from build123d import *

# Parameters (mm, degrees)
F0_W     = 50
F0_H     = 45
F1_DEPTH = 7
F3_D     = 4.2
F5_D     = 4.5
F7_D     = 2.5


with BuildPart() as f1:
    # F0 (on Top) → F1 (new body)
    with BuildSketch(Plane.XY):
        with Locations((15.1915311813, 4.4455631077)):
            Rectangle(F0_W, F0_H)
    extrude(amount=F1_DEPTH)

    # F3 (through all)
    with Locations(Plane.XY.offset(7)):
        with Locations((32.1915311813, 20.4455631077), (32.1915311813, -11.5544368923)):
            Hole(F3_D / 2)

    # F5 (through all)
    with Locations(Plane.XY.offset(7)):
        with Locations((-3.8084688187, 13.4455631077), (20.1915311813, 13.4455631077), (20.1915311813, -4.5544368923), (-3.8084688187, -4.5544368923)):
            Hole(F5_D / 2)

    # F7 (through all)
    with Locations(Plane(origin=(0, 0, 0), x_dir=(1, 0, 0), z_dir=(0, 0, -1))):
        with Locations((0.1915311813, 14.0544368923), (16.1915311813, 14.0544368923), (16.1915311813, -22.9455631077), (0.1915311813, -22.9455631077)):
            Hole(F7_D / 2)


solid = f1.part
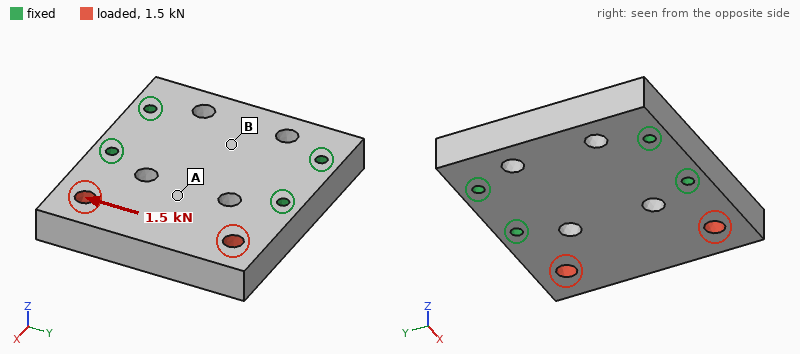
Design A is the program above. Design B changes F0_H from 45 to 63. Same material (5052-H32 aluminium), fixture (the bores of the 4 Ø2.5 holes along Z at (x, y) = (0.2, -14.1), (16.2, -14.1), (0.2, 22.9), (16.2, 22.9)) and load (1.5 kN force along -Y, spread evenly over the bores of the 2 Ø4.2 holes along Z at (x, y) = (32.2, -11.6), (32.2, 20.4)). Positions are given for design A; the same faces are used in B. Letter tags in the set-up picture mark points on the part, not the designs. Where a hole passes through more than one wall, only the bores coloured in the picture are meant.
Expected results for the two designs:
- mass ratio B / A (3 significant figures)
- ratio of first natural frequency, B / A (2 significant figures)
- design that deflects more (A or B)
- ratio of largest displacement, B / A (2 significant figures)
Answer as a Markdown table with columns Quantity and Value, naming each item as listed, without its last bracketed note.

| Quantity | Value |
|---|---|
| mass ratio B / A | 1.42 |
| ratio of first natural frequency, B / A | 1.0 |
| design that deflects more | A |
| ratio of largest displacement, B / A | 0.88 |
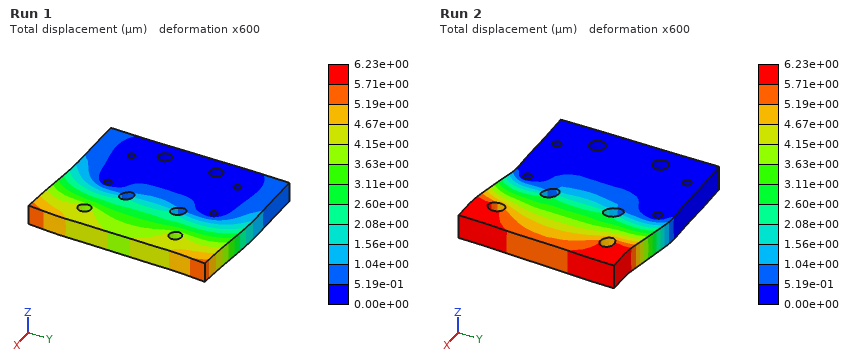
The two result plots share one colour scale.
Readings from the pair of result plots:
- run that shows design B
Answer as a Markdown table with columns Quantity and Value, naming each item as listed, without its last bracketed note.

| Quantity | Value |
|---|---|
| run that shows design B | Run 1 |
